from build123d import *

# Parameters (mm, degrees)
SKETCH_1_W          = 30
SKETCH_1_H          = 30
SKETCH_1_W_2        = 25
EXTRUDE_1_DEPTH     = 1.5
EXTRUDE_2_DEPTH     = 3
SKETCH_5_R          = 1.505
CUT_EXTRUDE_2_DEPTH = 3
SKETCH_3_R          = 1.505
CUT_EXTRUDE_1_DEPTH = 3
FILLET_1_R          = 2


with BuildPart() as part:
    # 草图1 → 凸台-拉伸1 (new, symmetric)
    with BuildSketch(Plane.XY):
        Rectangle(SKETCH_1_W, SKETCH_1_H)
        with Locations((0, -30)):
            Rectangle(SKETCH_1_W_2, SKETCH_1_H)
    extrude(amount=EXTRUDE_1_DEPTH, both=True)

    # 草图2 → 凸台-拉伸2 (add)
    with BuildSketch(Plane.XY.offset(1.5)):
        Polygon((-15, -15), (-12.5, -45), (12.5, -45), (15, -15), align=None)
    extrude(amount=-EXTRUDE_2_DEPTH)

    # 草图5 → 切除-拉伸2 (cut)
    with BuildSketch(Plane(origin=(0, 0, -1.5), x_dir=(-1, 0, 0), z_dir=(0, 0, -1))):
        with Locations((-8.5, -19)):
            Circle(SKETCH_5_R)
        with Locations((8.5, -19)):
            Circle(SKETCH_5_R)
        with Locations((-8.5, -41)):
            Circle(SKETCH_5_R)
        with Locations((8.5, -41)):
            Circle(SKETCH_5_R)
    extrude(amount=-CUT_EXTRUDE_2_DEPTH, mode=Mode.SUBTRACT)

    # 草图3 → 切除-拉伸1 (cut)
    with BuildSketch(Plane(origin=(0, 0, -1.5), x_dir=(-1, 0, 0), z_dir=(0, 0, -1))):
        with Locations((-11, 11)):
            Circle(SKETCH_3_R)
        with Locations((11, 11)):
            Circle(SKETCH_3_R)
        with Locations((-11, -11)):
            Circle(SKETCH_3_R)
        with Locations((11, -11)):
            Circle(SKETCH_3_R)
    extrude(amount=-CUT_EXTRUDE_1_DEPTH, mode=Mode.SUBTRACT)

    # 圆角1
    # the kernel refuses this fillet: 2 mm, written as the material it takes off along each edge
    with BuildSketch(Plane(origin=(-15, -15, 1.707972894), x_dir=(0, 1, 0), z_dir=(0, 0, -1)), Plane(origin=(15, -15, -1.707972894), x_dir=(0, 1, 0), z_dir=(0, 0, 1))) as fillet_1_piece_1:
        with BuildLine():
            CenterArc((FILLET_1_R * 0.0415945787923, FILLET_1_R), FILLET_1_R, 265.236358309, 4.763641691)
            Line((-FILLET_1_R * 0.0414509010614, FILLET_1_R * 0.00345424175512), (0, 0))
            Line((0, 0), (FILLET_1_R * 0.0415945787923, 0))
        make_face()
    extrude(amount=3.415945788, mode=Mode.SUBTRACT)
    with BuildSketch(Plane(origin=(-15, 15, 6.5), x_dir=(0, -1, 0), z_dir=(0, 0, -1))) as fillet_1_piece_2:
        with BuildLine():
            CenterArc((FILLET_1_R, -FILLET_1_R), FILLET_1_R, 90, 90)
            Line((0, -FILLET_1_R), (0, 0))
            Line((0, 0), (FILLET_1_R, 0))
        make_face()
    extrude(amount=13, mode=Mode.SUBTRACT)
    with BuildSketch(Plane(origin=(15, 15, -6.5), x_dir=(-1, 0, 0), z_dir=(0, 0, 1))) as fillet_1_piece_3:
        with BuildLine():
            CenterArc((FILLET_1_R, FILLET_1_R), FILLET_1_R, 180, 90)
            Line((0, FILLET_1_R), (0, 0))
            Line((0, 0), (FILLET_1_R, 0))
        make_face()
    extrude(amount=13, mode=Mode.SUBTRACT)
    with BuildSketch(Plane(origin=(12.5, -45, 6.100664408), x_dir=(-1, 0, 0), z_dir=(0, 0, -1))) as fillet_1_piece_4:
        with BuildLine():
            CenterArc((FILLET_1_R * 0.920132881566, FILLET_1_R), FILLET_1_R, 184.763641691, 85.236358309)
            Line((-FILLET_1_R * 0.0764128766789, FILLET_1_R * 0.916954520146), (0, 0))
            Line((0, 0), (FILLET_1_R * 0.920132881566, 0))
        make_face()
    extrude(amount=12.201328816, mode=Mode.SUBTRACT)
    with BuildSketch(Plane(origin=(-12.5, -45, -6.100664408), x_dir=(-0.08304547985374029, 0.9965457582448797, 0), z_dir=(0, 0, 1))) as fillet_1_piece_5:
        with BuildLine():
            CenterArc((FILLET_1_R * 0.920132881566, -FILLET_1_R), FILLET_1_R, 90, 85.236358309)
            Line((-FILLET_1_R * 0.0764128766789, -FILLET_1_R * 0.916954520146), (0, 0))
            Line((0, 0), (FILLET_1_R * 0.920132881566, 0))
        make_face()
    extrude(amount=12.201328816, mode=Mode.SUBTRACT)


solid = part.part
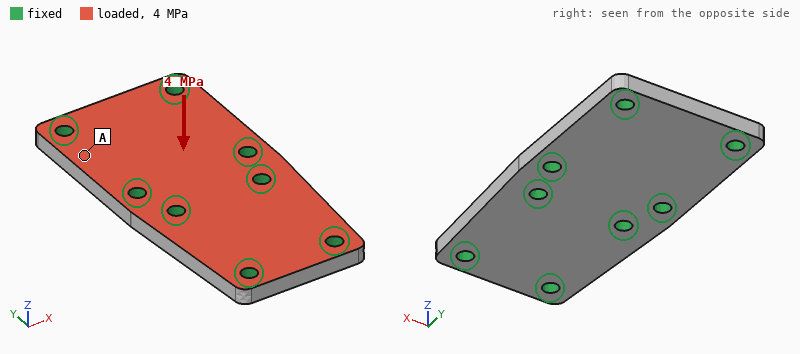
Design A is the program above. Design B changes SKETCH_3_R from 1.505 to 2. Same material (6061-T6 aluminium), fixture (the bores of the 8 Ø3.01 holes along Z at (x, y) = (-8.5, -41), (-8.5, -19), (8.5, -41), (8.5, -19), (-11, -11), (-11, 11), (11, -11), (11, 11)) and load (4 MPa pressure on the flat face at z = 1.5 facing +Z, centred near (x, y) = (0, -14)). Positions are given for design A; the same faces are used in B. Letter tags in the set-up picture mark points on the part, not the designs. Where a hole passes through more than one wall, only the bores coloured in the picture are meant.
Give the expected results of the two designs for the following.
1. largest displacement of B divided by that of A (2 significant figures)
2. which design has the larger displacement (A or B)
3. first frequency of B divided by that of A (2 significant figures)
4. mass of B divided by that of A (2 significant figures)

0.84
A
1.1
0.99
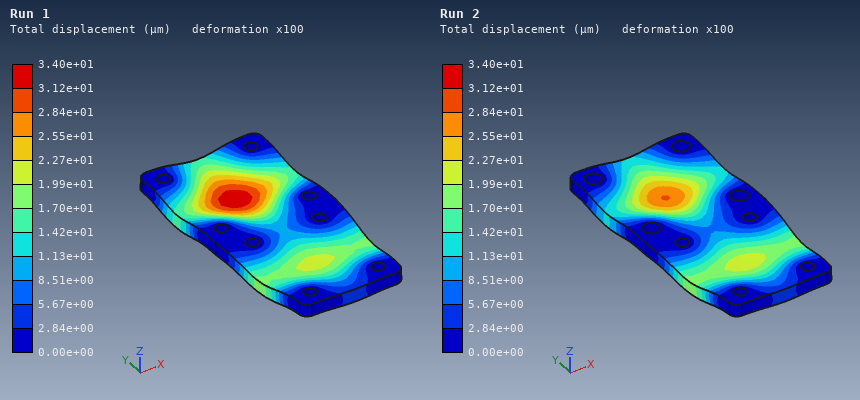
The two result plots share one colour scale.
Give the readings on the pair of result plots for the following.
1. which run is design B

Run 2
